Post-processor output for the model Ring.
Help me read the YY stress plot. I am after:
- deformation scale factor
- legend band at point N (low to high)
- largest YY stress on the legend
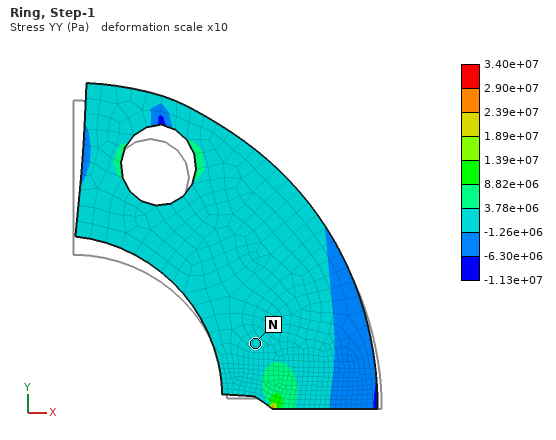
10
-1.26e+06 to 3.78e+06 Pa
3.40e+07 Pa
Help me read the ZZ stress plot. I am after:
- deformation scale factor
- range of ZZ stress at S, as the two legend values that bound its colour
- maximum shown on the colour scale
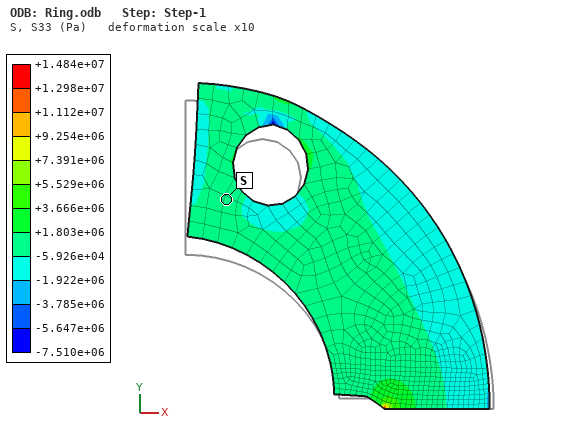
10
-5.926e+04 to +1.803e+06 Pa
+1.484e+07 Pa
